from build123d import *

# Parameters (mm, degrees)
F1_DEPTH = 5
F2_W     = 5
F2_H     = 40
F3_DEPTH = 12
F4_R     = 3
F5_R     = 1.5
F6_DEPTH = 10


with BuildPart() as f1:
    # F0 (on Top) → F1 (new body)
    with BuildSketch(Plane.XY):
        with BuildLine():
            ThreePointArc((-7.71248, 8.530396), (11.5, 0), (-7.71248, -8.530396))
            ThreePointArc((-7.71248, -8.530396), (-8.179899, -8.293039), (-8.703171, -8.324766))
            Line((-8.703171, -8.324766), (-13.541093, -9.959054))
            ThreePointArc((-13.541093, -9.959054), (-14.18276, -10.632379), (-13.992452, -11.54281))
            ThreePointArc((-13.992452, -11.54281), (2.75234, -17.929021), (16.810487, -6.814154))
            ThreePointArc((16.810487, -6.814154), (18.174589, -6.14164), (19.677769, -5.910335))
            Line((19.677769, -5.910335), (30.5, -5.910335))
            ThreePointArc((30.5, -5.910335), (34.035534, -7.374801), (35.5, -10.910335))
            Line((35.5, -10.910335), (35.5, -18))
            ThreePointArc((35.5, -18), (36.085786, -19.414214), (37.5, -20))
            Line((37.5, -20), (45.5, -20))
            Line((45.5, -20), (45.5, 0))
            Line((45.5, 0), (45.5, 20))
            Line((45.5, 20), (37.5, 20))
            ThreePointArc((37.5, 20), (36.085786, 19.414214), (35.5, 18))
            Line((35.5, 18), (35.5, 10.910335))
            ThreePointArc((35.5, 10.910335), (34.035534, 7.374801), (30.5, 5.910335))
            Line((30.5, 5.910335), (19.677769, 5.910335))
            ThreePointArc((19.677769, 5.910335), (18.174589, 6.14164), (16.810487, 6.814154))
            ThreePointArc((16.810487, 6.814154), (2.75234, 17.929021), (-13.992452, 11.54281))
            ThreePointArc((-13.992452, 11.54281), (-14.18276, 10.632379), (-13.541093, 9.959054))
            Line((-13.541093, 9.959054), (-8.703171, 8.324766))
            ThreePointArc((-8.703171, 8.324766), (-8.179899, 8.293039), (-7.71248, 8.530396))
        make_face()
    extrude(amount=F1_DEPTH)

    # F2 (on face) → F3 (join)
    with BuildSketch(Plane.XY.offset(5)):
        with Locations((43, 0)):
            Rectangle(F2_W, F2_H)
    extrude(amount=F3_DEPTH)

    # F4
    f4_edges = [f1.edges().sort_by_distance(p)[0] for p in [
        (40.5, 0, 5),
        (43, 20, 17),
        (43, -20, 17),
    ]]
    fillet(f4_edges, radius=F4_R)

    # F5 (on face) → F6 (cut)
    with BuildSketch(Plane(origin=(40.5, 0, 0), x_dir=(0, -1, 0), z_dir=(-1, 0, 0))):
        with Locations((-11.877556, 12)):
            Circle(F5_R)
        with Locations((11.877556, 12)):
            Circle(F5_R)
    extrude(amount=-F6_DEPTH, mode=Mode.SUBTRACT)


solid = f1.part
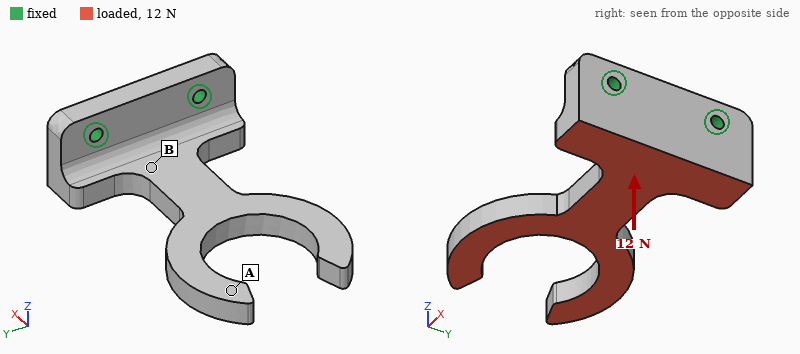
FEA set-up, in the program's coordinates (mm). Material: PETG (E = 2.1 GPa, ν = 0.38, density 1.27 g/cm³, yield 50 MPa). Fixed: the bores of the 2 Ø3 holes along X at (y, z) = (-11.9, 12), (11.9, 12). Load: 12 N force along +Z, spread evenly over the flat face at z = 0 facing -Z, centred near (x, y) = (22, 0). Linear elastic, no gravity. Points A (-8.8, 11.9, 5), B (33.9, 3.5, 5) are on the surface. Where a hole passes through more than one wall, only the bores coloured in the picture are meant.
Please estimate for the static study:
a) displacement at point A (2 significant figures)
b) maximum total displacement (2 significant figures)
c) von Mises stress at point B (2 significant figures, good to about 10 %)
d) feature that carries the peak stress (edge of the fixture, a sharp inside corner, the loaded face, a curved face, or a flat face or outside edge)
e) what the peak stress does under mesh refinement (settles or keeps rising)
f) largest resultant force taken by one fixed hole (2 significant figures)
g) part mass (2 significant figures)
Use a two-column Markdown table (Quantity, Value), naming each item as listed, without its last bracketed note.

| Quantity | Value |
|---|---|
| displacement at point A | 0.64 mm |
| maximum total displacement | 0.73 mm |
| von Mises stress at point B | 3.0 MPa |
| feature that carries the peak stress | edge of the fixture |
| what the peak stress does under mesh refinement | keeps rising |
| largest resultant force taken by one fixed hole | 7.0 N |
| part mass | 10 g |
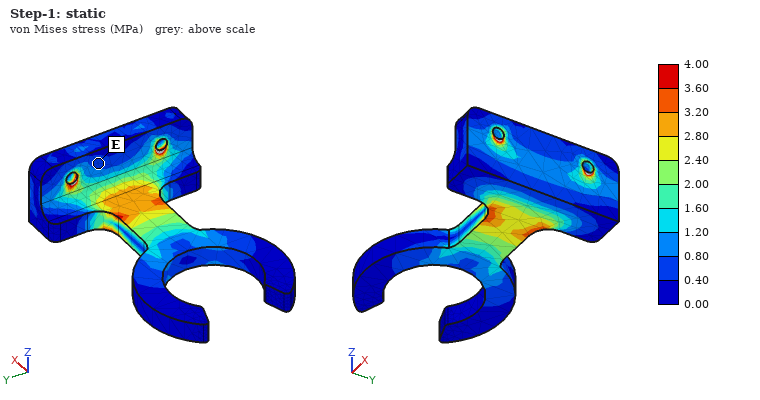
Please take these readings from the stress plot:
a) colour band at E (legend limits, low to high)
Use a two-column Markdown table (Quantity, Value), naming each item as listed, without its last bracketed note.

| Quantity | Value |
|---|---|
| colour band at E | 0.40 to 0.80 MPa |
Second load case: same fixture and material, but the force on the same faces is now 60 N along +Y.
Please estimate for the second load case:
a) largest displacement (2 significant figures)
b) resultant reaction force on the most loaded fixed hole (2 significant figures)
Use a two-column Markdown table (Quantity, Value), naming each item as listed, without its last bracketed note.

| Quantity | Value |
|---|---|
| largest displacement | 0.75 mm |
| resultant reaction force on the most loaded fixed hole | 64 N |
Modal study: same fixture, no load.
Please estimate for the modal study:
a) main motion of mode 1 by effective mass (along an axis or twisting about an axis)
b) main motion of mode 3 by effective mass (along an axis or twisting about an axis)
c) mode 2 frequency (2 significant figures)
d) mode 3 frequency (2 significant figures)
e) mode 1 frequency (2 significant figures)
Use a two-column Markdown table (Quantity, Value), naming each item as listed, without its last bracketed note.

| Quantity | Value |
|---|---|
| main motion of mode 1 by effective mass | along Z |
| main motion of mode 3 by effective mass | along Y |
| mode 2 frequency | 630 Hz |
| mode 3 frequency | 670 Hz |
| mode 1 frequency | 310 Hz |
